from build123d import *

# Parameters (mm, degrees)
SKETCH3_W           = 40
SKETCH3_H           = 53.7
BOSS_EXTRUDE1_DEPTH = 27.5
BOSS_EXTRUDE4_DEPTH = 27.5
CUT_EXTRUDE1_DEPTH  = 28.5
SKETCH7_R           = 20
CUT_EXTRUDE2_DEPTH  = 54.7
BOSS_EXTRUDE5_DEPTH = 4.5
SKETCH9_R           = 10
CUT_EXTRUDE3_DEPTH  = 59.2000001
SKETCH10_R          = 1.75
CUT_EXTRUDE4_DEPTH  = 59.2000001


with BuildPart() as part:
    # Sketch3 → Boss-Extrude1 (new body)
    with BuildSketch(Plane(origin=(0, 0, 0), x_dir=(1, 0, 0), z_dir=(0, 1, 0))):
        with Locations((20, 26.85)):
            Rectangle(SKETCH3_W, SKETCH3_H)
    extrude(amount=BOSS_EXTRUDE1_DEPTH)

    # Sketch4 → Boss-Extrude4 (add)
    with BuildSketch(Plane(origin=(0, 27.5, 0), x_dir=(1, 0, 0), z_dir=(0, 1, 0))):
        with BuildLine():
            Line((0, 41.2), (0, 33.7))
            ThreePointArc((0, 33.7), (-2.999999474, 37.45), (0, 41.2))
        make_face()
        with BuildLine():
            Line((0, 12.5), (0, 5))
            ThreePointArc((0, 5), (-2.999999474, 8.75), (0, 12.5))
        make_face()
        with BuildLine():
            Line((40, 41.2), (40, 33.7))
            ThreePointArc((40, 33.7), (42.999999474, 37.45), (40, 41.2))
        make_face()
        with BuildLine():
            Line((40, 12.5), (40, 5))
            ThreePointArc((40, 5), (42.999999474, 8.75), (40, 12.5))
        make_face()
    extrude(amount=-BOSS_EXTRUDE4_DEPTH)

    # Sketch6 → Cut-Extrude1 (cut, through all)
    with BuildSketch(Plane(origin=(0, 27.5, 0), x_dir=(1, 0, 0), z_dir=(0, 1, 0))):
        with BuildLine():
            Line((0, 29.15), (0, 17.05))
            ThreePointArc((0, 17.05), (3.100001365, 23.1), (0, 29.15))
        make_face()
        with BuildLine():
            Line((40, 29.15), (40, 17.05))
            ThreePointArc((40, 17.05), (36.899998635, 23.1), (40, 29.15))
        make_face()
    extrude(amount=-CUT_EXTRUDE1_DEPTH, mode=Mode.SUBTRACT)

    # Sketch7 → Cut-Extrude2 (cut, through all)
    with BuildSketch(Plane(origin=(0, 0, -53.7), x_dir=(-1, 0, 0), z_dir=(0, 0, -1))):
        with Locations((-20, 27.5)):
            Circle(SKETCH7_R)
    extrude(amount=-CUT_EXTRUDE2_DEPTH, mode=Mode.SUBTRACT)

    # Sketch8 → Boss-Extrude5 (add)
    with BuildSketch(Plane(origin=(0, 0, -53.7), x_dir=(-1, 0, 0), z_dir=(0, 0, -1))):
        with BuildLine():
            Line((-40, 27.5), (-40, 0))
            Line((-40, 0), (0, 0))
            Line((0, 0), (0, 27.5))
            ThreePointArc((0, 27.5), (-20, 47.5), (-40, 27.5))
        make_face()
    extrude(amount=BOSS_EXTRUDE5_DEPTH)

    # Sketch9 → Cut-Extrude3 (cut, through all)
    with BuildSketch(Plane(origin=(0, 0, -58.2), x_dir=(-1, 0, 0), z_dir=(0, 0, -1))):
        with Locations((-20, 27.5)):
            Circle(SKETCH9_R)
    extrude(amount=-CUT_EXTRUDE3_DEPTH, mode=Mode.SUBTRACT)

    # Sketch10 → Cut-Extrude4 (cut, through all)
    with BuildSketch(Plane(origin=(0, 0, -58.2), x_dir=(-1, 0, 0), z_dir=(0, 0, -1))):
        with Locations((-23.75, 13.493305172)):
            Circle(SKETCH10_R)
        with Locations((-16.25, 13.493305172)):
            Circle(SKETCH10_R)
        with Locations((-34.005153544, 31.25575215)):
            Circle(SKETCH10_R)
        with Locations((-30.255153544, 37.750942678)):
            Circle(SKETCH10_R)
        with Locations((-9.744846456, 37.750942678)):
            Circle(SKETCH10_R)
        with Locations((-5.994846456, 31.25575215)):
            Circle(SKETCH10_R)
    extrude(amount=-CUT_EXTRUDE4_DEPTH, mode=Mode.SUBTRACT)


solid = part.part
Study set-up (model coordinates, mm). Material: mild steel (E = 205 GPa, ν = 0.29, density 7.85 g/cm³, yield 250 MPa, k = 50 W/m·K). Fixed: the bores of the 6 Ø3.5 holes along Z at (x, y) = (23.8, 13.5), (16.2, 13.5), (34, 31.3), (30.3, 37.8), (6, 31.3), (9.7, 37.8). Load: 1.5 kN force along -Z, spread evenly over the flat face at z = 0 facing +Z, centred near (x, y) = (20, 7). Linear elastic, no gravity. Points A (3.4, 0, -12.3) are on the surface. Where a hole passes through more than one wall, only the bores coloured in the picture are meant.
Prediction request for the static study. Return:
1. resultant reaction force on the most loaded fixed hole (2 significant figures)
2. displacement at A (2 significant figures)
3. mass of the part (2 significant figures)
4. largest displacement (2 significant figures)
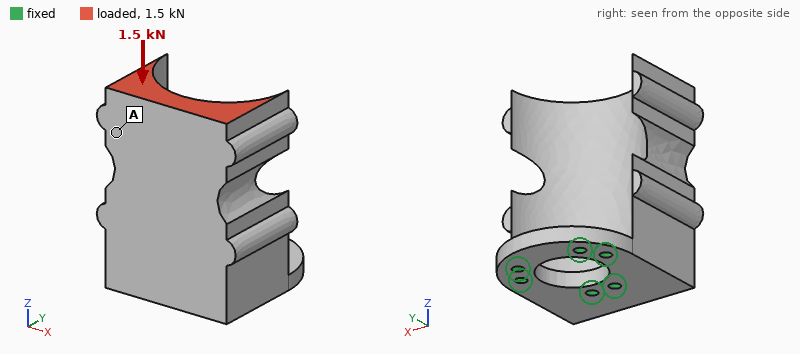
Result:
850 N
16 µm
250 g
19 µm
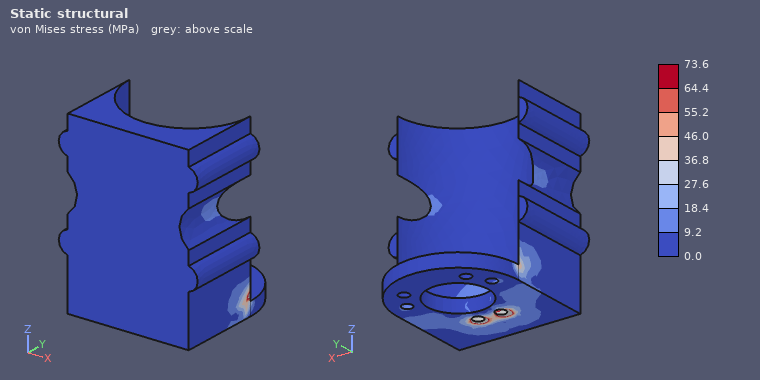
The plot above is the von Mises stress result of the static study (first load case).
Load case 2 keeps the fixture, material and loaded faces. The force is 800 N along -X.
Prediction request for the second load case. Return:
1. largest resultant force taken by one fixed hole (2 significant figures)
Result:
1.6 kN
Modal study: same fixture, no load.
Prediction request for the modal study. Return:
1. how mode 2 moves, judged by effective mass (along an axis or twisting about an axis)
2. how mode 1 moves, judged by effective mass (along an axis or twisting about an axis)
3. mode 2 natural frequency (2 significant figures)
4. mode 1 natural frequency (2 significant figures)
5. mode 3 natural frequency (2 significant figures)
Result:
along X
along Y
1900 Hz
1500 Hz
5000 Hz
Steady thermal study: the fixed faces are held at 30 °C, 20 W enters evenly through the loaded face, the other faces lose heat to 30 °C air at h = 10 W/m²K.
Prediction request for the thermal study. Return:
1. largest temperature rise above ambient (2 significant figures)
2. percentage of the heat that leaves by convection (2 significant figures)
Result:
60 K
17 %
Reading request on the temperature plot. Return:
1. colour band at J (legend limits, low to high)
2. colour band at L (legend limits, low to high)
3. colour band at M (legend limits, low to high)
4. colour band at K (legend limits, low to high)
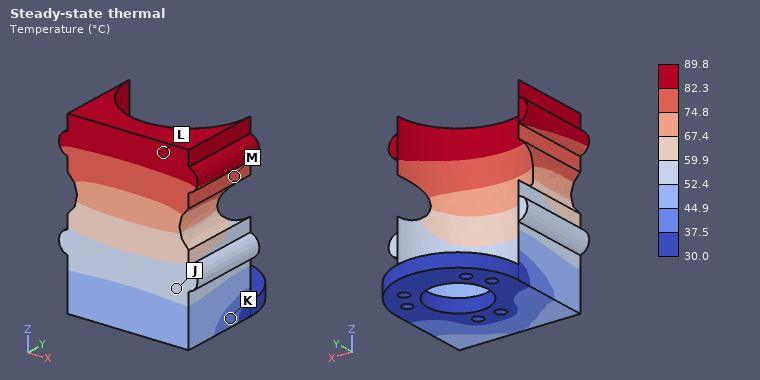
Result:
52.4 to 59.9 °C
82.3 to 89.8 °C
74.8 to 82.3 °C
37.5 to 44.9 °C
